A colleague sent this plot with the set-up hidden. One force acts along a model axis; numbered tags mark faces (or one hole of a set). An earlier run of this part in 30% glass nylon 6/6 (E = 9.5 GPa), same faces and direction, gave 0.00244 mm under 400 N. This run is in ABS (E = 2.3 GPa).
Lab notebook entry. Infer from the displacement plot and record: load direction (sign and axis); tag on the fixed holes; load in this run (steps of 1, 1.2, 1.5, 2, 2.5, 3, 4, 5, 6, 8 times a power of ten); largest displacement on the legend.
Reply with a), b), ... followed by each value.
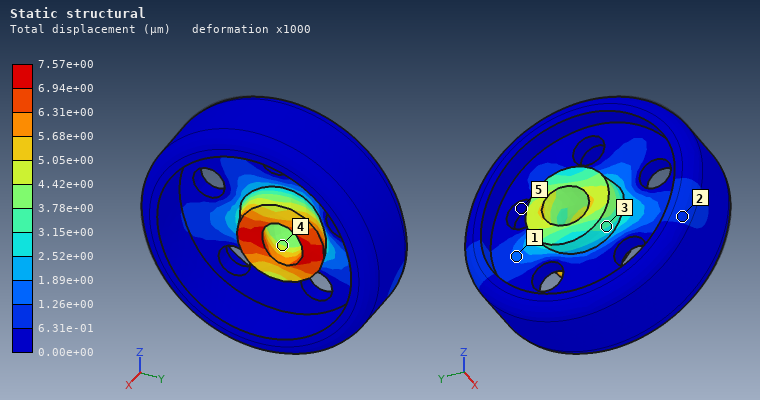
a) +Y
b) 5
c) 300 N
d) 7.57e+00 µm
